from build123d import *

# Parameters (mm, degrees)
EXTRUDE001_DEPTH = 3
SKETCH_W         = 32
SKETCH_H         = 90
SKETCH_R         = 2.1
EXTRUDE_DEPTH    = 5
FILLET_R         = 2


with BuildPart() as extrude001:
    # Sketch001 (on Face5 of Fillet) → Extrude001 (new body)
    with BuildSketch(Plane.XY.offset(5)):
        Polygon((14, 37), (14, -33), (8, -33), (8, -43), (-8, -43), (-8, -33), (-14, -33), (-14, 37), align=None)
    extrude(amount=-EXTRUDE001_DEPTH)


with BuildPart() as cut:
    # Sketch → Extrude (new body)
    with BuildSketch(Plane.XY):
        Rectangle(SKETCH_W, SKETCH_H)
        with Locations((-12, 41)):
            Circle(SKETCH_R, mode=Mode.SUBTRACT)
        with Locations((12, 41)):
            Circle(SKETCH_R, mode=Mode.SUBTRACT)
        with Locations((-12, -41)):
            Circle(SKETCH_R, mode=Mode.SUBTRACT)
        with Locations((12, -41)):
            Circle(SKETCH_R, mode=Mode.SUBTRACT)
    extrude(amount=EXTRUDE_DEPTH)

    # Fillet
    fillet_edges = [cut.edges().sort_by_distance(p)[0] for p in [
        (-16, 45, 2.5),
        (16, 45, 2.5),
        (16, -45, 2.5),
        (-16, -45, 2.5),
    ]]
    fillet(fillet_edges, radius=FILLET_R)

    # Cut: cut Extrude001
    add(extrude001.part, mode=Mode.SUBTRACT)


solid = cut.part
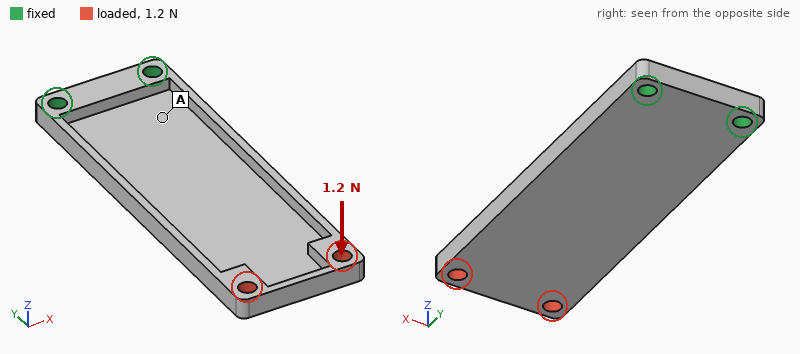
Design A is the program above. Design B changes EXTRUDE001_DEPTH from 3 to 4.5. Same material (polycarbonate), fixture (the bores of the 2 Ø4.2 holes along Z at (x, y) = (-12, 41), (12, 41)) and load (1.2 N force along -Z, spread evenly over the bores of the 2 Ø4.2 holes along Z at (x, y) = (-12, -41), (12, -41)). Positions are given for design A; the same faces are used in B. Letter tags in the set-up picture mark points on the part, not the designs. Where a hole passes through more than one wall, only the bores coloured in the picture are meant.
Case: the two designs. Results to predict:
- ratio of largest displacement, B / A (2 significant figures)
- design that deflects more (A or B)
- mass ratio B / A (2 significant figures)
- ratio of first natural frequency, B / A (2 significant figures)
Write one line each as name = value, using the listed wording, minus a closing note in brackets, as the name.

ratio of largest displacement, B / A = 1.1
design that deflects more = B
mass ratio B / A = 0.59
ratio of first natural frequency, B / A = 1.1
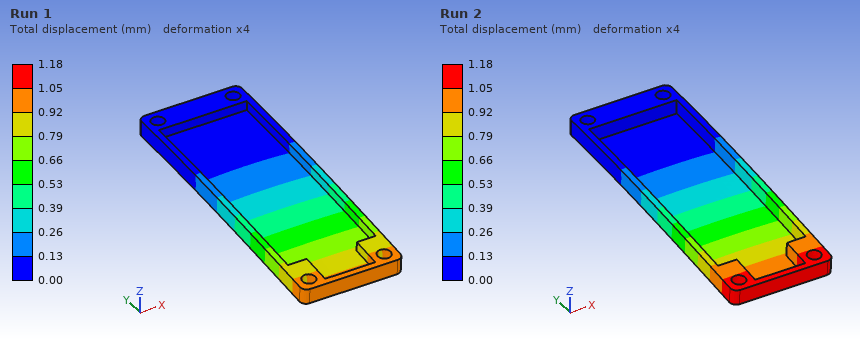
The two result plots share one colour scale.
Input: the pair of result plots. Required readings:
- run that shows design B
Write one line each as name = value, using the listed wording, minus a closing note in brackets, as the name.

run that shows design B = Run 2
